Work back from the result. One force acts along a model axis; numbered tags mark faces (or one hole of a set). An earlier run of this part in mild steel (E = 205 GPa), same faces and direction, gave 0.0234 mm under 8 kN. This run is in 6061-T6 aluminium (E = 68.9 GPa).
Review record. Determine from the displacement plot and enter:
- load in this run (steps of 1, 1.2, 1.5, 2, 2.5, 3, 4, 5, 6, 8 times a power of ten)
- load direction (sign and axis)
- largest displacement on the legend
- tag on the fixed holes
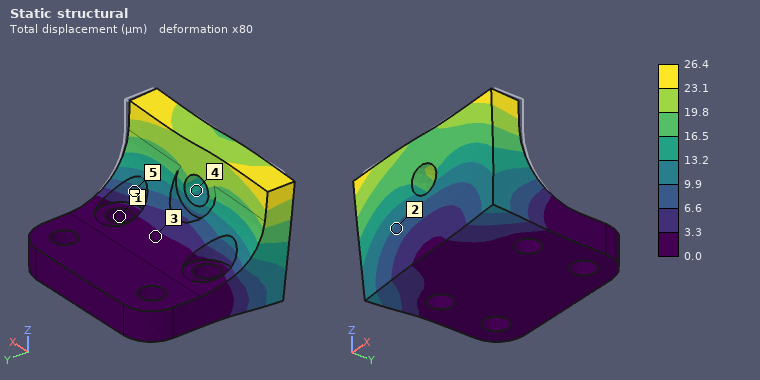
3 kN
-X
26.4 µm
1
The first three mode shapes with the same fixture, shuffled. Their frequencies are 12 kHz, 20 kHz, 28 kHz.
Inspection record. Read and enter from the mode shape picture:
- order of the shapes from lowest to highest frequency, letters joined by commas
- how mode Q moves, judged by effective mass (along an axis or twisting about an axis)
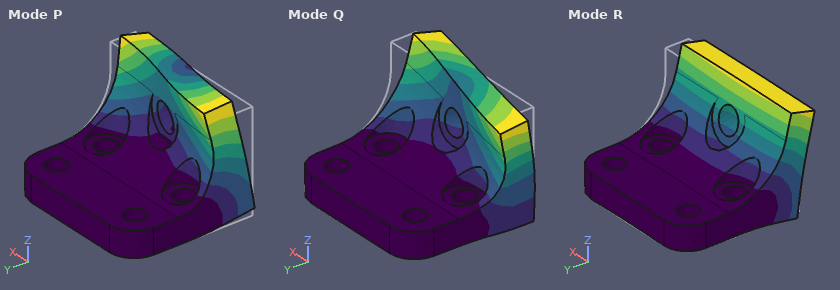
R, P, Q
along X
